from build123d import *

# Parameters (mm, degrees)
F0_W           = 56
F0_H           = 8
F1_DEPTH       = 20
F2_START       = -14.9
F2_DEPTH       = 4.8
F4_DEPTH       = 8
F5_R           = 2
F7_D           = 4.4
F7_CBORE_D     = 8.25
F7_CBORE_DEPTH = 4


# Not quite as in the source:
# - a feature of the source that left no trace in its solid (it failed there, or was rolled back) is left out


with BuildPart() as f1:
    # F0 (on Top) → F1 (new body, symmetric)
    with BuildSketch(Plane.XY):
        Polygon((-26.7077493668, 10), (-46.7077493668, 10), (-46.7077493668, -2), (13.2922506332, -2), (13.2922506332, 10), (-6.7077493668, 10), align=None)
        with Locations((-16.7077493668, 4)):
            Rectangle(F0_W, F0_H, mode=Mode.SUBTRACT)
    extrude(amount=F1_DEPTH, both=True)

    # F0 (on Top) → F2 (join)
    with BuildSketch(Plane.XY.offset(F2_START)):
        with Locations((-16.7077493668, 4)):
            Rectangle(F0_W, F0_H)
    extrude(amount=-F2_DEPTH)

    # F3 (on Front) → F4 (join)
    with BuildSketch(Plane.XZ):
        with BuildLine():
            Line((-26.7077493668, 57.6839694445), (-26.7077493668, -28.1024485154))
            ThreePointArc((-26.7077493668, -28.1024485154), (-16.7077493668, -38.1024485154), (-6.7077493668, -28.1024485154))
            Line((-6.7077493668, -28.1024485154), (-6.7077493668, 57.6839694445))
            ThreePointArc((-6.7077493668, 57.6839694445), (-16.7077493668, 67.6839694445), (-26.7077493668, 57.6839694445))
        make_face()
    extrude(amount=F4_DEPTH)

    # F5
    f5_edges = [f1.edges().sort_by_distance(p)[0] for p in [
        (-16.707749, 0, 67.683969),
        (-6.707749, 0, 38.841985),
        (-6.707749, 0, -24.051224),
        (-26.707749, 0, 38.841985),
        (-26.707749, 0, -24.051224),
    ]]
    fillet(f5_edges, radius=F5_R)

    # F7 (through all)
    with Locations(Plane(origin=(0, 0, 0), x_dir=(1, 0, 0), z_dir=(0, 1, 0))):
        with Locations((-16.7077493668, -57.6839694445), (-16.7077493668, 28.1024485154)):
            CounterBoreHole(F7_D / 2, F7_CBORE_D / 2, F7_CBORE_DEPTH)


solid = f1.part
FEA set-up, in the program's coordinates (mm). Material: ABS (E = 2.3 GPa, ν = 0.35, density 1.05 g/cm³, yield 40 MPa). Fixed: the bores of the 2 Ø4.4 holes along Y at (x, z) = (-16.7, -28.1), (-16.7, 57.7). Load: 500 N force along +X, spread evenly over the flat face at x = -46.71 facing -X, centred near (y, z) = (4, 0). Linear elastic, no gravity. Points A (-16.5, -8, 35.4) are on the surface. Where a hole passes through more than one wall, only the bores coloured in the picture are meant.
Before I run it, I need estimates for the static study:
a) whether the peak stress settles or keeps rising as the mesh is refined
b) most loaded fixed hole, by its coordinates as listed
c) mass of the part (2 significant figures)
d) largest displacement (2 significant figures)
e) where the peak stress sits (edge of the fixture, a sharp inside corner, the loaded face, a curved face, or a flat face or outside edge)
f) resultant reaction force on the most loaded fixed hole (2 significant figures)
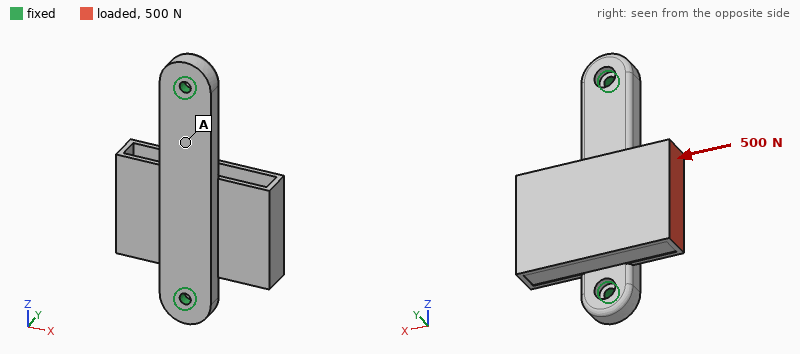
keeps rising
(-16.7, -28.1)
28 g
1.4 mm
edge of the fixture
340 N
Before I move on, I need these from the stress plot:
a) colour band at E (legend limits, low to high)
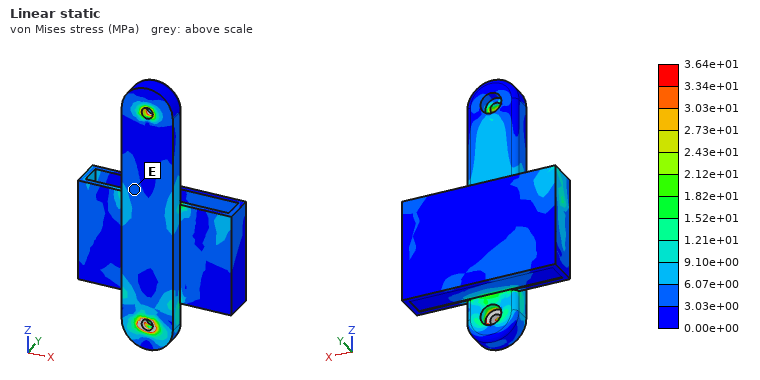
3.03e+00 to 6.07e+00 MPa
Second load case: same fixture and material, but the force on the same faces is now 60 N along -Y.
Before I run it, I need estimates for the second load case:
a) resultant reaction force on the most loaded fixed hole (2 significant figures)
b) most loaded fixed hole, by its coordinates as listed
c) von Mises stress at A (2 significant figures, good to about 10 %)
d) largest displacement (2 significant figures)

64 N
(-16.7, -28.1)
2.4 MPa
1.0 mm
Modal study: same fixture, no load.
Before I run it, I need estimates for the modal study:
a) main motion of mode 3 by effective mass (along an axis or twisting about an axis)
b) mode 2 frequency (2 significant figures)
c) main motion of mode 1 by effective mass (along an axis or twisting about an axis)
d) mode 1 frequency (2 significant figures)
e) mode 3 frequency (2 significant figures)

along Y
670 Hz
along Y
630 Hz
1300 Hz
